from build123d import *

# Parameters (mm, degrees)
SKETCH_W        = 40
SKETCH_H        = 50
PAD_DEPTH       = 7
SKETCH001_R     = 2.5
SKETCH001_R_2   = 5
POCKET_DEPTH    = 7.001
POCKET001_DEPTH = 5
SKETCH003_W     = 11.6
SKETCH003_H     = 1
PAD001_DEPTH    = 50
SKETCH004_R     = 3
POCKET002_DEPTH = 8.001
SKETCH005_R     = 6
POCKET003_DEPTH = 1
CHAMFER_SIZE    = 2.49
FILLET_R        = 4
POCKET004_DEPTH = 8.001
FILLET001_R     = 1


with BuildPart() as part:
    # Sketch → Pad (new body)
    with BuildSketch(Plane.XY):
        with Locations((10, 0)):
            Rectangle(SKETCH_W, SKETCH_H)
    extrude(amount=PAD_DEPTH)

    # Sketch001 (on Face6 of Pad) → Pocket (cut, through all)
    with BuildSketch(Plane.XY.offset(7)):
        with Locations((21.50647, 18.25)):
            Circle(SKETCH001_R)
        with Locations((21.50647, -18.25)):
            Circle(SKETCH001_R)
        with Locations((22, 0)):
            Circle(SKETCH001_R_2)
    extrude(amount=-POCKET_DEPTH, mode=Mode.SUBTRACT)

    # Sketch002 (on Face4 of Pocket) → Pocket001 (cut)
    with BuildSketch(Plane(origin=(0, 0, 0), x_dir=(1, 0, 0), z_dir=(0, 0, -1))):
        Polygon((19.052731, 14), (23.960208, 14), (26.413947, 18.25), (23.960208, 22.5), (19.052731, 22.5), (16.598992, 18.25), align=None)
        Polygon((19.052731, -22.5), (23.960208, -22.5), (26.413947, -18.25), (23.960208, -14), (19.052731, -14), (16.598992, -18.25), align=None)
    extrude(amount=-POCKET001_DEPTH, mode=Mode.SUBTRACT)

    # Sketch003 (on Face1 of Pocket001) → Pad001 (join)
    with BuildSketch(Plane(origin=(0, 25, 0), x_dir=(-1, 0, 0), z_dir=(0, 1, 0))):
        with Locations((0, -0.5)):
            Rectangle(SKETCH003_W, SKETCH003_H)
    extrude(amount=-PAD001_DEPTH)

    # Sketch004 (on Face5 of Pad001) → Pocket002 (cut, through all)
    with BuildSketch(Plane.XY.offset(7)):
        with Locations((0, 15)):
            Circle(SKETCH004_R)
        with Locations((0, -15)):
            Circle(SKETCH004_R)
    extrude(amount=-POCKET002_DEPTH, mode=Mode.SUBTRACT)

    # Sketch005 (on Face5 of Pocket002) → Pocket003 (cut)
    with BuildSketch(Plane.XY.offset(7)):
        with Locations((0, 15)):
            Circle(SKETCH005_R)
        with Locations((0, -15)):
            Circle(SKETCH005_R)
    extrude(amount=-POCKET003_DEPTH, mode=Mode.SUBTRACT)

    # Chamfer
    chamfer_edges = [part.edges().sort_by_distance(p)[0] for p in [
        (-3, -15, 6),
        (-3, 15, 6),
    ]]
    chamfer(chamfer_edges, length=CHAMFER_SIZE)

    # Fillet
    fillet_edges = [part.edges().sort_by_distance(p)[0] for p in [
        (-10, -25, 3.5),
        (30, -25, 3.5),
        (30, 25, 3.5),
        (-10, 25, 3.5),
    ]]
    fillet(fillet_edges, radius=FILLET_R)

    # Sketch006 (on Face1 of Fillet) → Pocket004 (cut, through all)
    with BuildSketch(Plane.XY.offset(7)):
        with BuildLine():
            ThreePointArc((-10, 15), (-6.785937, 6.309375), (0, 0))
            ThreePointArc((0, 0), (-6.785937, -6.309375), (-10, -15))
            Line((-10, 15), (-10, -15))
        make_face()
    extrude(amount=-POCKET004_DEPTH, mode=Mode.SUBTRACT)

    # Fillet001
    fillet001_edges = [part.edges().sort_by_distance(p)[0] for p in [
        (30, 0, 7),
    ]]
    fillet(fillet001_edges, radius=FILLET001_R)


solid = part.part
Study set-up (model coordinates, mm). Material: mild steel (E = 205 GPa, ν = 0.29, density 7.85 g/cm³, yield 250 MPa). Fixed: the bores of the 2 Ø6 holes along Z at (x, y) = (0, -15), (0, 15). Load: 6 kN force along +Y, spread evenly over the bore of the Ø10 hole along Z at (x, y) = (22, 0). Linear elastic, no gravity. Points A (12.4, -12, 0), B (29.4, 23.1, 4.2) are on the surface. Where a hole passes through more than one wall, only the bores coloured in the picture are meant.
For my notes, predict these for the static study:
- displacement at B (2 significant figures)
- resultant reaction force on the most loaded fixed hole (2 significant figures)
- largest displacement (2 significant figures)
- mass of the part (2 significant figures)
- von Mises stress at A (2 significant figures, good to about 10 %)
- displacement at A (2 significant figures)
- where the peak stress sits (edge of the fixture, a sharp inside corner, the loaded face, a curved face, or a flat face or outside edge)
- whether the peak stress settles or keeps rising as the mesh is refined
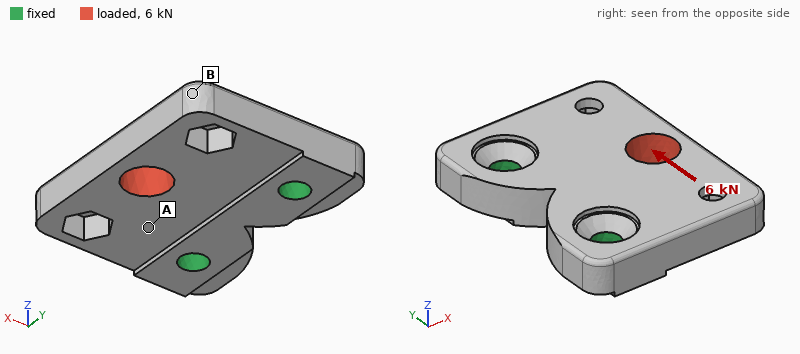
15 µm
4.8 kN
15 µm
92 g
43 MPa
5.1 µm
edge of the fixture
keeps rising
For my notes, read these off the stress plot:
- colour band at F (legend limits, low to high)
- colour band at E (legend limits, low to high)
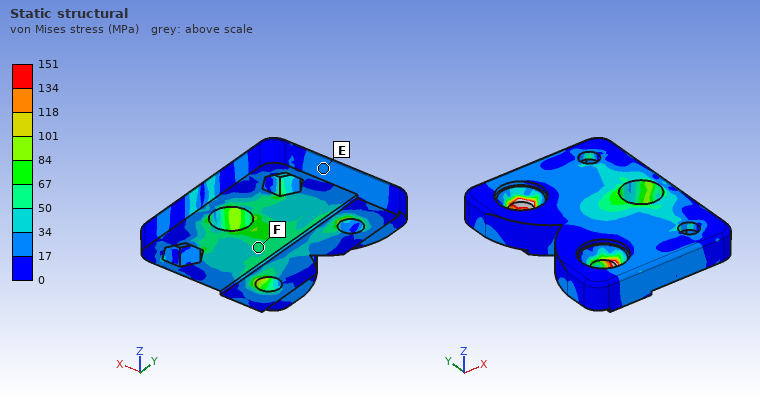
50 to 67 MPa
17 to 34 MPa
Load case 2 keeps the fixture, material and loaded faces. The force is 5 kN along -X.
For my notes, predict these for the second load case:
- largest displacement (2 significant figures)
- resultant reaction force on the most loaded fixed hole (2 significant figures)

11 µm
2.7 kN
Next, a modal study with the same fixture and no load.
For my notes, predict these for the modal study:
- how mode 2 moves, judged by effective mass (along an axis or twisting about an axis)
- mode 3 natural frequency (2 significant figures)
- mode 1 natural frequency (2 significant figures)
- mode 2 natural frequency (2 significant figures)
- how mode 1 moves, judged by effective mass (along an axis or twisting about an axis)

twisting about X
18 kHz
5700 Hz
9600 Hz
along Z
